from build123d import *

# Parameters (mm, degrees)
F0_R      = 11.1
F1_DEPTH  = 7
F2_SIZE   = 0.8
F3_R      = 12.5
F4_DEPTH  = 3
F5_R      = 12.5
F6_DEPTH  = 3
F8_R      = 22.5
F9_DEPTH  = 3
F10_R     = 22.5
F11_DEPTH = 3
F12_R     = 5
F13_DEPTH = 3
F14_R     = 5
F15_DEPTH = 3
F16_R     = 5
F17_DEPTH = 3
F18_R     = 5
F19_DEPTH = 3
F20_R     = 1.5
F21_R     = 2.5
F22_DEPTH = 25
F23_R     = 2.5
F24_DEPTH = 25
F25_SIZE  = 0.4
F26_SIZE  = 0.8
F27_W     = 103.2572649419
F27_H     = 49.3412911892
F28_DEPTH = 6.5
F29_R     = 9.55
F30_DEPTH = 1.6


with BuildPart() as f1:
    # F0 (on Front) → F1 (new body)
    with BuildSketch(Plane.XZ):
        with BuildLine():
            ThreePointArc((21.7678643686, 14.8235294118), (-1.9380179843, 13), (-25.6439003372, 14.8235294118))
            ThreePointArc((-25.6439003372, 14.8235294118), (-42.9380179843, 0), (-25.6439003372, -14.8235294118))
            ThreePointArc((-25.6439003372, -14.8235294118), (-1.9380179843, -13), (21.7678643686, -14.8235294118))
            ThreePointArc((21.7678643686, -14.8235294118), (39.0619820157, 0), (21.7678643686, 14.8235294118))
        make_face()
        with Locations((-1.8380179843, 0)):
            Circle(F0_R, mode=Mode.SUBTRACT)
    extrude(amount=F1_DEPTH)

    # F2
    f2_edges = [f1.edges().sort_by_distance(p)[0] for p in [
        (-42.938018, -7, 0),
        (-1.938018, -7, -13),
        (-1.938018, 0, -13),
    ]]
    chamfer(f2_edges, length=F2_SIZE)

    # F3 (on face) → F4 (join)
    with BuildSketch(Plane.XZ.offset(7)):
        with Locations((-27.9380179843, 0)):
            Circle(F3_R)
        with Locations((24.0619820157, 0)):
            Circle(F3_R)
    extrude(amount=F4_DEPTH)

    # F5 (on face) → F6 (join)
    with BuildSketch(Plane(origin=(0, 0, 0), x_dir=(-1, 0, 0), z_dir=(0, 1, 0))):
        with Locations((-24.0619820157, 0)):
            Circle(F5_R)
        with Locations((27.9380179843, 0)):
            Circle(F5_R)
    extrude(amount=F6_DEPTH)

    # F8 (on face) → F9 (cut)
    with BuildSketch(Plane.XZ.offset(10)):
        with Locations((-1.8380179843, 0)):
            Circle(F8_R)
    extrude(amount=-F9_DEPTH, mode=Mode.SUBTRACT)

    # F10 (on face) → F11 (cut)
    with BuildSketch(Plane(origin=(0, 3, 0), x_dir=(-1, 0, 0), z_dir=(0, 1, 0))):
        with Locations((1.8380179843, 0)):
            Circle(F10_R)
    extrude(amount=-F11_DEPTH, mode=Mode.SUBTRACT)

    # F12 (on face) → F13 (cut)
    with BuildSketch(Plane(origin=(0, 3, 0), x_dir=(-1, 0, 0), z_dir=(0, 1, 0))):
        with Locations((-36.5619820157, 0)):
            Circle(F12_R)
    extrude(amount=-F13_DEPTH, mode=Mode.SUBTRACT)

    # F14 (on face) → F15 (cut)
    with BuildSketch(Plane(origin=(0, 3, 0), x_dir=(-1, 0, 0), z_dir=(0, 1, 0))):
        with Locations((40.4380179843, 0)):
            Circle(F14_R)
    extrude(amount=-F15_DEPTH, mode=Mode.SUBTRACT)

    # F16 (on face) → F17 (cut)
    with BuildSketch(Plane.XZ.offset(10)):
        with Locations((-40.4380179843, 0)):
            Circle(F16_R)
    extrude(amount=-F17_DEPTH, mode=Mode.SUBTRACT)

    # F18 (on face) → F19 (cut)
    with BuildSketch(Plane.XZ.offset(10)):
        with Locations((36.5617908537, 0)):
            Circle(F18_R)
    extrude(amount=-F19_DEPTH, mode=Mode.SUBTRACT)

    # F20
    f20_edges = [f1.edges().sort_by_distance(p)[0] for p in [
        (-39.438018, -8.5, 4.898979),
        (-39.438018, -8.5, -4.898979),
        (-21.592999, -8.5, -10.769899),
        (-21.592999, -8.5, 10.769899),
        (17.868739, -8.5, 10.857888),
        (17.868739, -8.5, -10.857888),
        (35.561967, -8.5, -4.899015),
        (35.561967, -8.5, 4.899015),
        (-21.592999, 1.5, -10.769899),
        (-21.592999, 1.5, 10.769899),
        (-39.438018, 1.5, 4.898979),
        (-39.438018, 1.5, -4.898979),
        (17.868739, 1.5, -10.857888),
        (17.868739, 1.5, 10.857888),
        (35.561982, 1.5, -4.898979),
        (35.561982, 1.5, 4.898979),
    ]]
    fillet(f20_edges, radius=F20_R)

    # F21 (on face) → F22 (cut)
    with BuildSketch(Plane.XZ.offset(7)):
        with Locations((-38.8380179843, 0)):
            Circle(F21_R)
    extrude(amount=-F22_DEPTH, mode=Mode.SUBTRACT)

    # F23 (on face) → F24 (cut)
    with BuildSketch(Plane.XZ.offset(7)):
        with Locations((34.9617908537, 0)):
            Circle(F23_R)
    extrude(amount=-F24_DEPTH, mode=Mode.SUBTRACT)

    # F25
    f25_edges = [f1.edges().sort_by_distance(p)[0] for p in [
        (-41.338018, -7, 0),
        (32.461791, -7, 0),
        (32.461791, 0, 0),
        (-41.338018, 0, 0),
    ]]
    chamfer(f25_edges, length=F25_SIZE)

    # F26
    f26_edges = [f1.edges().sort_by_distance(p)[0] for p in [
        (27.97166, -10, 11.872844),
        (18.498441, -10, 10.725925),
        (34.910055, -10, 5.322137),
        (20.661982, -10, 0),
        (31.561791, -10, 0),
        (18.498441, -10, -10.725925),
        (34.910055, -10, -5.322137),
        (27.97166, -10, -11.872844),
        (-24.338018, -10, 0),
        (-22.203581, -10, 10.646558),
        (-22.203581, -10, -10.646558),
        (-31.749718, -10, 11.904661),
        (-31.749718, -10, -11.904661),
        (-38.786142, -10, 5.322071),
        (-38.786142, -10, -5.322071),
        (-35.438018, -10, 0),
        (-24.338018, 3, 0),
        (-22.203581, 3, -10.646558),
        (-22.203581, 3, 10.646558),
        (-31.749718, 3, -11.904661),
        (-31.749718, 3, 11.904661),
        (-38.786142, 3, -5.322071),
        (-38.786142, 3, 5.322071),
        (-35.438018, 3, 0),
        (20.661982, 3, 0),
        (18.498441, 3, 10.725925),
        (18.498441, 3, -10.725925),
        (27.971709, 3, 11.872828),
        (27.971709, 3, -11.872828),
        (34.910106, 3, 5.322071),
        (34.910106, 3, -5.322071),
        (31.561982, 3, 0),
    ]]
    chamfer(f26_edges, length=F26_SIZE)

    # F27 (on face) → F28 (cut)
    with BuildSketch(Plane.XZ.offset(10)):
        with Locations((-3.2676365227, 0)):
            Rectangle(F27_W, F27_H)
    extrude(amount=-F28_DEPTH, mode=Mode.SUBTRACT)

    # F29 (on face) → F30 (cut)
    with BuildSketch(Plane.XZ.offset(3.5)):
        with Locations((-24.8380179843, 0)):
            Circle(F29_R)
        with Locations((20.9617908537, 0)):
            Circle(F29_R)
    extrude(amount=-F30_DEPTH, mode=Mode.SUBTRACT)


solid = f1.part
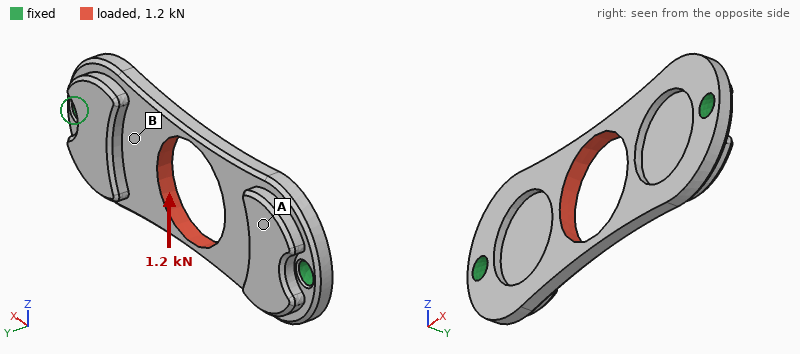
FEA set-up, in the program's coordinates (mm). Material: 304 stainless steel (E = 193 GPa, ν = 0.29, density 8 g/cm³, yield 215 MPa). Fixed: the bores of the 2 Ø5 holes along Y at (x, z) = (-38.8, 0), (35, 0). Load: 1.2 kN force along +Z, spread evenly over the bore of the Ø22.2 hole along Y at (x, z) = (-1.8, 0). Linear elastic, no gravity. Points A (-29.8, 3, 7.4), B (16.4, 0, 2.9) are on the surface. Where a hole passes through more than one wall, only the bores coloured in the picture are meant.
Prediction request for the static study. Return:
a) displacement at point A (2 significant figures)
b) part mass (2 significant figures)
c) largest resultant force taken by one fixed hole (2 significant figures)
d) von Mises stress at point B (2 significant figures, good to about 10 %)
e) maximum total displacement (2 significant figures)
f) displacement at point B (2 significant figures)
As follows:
4.6 µm
55 g
600 N
19 MPa
21 µm
8.0 µm
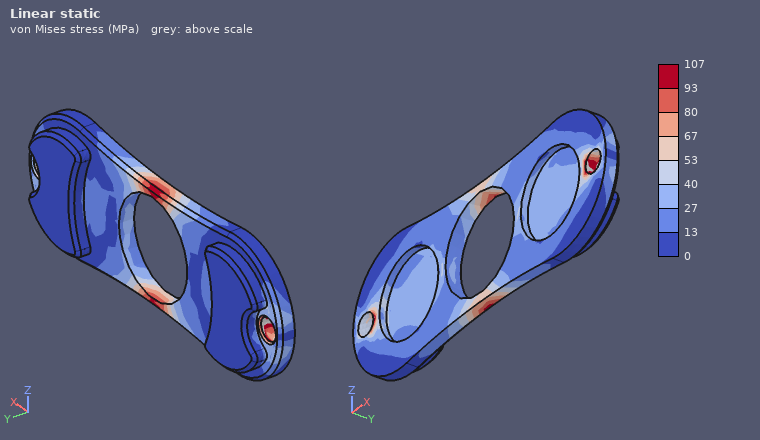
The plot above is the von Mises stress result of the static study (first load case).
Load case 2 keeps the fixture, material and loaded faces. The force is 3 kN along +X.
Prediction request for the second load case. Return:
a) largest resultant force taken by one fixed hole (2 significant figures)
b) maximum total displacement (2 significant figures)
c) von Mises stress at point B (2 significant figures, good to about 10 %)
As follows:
1.5 kN
5.8 µm
23 MPa
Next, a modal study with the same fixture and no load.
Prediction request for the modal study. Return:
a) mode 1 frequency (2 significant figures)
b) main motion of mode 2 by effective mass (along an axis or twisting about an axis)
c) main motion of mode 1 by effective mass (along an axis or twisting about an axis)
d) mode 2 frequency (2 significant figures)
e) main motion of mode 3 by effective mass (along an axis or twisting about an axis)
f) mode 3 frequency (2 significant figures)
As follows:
3900 Hz
twisting about X
along Y
5900 Hz
twisting about Z
7100 Hz
